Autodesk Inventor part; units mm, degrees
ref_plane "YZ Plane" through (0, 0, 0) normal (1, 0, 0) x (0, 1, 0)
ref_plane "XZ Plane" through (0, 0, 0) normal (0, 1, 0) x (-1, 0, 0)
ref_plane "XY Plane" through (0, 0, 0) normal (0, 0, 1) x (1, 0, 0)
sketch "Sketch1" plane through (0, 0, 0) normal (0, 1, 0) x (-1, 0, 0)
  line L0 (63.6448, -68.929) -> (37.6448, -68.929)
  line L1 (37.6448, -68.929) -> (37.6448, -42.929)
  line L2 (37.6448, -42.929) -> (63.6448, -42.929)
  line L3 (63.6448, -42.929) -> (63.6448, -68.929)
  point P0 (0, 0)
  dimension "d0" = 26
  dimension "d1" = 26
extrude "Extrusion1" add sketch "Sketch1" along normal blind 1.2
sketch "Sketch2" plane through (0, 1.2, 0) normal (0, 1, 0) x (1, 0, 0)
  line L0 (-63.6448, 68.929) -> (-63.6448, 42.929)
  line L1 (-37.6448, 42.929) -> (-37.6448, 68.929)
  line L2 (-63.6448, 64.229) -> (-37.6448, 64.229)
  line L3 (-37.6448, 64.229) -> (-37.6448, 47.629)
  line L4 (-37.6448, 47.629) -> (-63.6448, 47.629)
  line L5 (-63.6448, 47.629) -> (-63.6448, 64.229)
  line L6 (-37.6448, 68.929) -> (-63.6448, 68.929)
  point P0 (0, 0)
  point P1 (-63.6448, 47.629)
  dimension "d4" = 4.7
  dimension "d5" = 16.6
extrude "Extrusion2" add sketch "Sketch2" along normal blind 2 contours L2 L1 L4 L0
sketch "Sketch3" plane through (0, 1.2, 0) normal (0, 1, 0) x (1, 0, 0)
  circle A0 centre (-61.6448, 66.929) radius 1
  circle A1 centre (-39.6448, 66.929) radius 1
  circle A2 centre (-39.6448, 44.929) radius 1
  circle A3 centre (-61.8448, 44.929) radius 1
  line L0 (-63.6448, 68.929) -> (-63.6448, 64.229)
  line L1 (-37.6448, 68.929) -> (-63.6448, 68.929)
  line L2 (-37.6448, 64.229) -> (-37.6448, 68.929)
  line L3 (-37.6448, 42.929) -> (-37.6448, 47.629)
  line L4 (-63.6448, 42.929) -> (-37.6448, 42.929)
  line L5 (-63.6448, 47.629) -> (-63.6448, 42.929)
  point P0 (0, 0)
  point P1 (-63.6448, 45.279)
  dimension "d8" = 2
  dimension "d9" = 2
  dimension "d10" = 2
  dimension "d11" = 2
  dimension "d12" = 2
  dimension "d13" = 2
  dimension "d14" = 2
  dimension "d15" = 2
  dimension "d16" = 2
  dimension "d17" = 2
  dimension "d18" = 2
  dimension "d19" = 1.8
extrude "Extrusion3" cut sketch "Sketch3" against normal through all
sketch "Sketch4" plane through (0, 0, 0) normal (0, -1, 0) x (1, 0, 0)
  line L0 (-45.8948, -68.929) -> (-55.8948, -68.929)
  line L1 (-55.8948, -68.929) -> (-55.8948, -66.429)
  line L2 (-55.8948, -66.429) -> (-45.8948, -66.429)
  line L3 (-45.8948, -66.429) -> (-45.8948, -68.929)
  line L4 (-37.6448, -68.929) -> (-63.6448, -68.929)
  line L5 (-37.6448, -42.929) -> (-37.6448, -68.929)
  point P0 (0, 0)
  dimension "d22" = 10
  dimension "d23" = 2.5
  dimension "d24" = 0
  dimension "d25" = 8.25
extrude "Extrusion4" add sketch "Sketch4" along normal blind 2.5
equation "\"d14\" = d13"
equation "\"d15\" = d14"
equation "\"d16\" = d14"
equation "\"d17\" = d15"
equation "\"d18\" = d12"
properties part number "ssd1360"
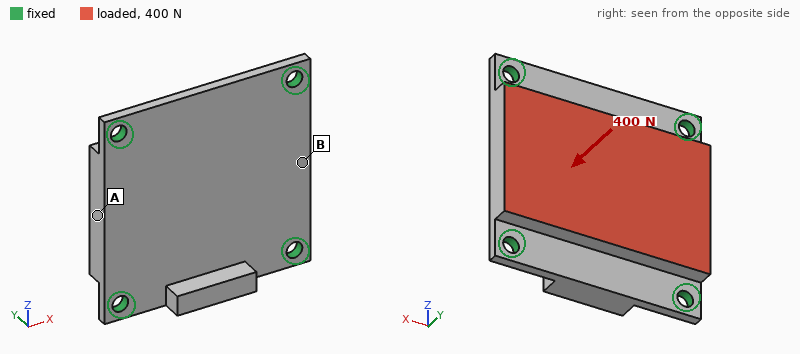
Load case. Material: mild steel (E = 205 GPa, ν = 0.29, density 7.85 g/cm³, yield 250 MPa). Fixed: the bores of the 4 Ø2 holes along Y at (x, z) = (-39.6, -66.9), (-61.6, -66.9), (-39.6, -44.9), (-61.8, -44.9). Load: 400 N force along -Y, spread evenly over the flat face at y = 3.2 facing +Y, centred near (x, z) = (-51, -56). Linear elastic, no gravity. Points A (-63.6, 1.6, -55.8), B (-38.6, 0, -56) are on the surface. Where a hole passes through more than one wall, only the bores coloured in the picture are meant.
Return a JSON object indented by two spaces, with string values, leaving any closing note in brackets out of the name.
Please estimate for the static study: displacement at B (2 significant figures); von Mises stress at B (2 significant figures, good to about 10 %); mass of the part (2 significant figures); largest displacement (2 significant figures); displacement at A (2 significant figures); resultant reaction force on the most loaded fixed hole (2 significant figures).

{
  "displacement at B": "3.3 µm",
  "von Mises stress at B": "17 MPa",
  "mass of the part": "14 g",
  "largest displacement": "5.4 µm",
  "displacement at A": "3.2 µm",
  "resultant reaction force on the most loaded fixed hole": "150 N"
}
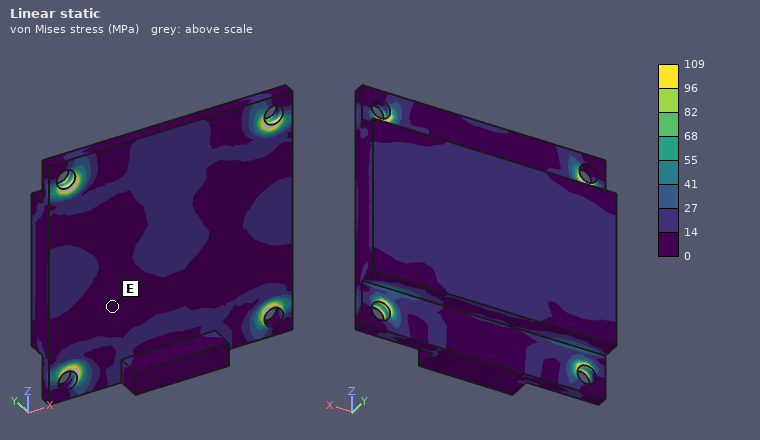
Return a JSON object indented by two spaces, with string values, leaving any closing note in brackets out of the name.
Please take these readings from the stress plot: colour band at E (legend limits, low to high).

{
  "colour band at E": "0 to 14 MPa"
}
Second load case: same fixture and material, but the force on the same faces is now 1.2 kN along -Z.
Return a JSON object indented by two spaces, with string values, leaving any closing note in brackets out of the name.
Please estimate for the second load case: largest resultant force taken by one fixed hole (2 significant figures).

{
  "largest resultant force taken by one fixed hole": "330 N"
}
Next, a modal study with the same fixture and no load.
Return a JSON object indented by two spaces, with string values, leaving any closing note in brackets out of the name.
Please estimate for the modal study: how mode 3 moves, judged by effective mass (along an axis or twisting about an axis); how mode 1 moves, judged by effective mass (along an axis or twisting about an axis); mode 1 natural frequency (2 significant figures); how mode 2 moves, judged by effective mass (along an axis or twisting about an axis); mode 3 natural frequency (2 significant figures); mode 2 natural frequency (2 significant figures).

{
  "how mode 3 moves, judged by effective mass": "twisting about Z",
  "how mode 1 moves, judged by effective mass": "along Y",
  "mode 1 natural frequency": "14 kHz",
  "how mode 2 moves, judged by effective mass": "twisting about X",
  "mode 3 natural frequency": "23 kHz",
  "mode 2 natural frequency": "20 kHz"
}
